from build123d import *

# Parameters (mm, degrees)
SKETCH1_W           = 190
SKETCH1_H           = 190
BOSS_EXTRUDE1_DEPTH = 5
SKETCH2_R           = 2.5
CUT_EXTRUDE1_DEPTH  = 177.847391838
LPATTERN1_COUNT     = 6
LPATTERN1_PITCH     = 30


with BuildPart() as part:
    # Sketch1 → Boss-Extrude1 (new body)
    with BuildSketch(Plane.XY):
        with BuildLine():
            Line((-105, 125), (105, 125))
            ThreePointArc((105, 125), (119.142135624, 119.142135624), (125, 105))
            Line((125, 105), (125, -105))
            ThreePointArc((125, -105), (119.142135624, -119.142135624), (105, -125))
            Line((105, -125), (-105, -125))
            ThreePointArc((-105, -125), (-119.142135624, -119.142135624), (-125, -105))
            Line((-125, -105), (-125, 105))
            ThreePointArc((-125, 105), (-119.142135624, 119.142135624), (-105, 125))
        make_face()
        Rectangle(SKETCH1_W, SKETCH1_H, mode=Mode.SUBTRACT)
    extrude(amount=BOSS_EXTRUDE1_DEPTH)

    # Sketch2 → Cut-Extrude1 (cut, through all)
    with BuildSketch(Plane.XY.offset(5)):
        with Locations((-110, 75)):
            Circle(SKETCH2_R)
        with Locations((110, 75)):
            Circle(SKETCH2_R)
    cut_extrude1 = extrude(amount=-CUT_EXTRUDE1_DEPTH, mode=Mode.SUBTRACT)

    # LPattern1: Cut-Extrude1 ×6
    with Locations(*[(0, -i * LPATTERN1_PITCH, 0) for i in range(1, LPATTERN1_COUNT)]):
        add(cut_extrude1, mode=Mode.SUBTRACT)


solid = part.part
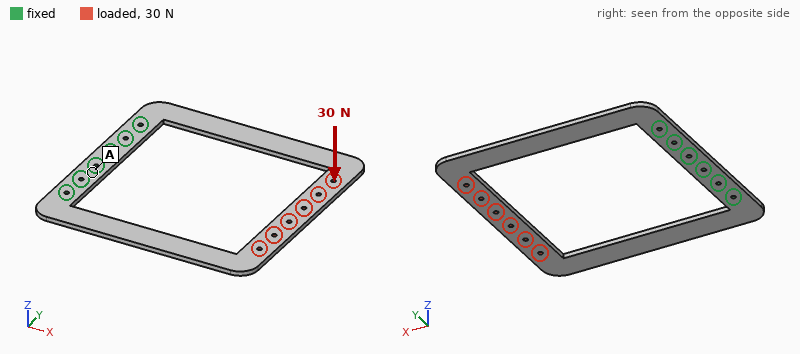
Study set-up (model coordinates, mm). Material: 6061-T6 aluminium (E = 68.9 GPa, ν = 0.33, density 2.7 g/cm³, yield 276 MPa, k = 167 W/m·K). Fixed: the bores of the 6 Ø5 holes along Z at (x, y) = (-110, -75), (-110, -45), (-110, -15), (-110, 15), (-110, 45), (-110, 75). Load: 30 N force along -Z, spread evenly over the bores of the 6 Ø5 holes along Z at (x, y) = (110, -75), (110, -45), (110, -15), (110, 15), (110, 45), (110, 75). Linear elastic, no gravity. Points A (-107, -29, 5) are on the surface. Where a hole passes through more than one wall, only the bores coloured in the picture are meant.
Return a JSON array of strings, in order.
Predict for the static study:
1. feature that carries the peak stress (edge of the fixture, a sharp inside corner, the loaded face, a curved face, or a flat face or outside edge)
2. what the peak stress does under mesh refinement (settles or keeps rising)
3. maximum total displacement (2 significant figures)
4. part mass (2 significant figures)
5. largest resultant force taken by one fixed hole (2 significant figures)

["edge of the fixture", "keeps rising", "3.4 mm", "350 g", "19 N"]
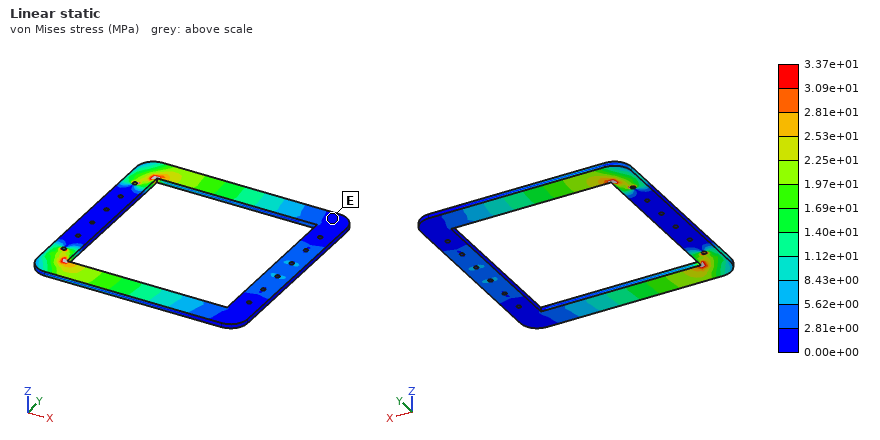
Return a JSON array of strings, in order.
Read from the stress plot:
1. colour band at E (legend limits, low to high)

["0.00e+00 to 2.81e+00 MPa"]
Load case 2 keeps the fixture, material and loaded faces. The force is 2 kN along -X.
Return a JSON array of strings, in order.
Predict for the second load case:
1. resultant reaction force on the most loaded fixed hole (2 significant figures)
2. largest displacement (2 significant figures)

["1.8 kN", "0.30 mm"]
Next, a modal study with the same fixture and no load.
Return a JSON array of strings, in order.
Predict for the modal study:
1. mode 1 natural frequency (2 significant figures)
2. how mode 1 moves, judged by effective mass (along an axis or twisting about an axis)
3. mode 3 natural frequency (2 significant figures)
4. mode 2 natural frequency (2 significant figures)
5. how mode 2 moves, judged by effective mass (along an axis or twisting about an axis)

["44 Hz", "along Z", "300 Hz", "100 Hz", "twisting about X"]
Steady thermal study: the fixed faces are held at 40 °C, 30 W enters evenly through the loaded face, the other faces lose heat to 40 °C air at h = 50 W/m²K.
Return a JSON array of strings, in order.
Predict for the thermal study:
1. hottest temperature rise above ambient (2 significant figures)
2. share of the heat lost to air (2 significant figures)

["32 K", "96 %"]
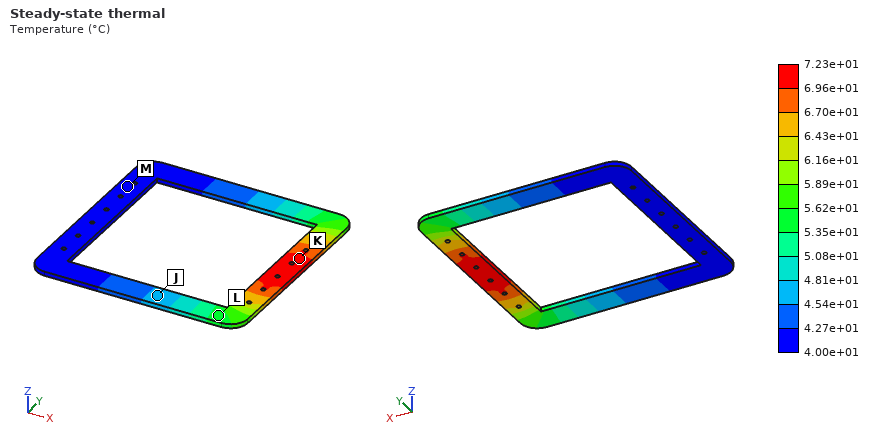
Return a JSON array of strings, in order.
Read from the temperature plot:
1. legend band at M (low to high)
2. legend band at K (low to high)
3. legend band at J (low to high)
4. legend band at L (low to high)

["4.00e+01 to 4.27e+01 °C", "6.96e+01 to 7.23e+01 °C", "4.54e+01 to 4.81e+01 °C", "5.35e+01 to 5.62e+01 °C"]
